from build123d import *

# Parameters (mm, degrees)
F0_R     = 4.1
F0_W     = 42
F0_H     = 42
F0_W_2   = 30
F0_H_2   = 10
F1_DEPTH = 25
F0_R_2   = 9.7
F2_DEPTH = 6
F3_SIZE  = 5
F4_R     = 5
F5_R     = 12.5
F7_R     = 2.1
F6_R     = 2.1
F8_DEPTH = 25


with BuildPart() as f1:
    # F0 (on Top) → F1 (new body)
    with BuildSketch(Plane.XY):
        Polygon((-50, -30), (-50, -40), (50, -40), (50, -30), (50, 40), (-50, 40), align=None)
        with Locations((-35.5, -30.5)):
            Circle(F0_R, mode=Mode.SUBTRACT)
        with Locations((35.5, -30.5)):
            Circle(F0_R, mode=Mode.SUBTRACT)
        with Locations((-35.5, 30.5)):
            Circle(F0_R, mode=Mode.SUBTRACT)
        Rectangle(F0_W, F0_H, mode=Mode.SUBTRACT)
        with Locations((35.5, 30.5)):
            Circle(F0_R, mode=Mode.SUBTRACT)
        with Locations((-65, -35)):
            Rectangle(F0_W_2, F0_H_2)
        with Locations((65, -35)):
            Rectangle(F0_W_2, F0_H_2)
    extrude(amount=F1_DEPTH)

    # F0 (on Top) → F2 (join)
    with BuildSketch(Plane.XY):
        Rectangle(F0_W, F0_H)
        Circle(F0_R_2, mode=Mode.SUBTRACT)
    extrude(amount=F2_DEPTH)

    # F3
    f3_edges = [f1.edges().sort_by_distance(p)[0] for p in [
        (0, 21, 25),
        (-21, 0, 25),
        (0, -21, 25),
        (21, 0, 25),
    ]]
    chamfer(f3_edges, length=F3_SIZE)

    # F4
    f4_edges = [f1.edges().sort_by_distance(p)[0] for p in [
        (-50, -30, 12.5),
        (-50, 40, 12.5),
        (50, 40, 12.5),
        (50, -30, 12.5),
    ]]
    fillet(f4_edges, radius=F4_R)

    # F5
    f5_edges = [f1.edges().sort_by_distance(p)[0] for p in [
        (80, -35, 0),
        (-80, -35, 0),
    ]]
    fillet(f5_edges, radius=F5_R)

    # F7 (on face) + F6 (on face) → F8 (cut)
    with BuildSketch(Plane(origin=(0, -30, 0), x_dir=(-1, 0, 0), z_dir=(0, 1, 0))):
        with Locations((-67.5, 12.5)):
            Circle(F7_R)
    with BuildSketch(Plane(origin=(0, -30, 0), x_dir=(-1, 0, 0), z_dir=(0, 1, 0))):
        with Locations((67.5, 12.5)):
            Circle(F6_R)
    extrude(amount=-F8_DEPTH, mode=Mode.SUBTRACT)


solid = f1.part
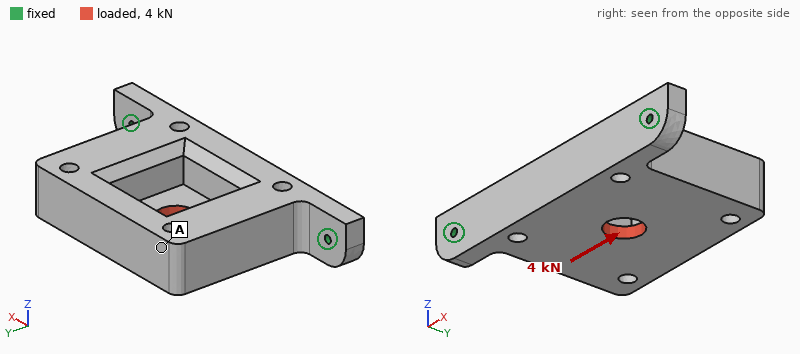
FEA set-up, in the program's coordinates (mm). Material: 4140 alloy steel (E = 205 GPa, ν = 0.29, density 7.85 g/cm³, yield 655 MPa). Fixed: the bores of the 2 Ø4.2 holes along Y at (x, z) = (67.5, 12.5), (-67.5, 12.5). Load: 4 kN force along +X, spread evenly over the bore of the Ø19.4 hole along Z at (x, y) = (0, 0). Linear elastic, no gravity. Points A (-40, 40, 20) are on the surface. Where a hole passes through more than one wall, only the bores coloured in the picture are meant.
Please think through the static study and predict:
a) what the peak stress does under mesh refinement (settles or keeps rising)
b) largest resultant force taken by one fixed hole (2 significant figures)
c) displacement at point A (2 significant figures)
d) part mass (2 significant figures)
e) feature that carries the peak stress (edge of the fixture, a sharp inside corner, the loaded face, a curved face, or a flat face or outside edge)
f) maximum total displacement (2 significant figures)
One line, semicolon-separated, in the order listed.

keeps rising; 2.3 kN; 8.0 µm; 1.3 kg; edge of the fixture; 8.9 µm
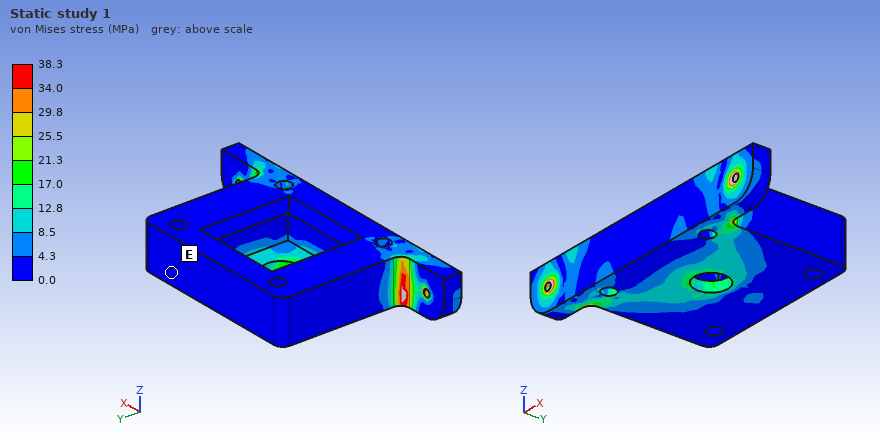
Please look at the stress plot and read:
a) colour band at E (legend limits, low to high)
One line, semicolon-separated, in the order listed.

0.0 to 4.3 MPa
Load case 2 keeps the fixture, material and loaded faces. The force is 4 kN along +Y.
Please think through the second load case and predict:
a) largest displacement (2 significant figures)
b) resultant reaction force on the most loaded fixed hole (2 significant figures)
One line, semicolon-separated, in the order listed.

64 µm; 2.3 kN
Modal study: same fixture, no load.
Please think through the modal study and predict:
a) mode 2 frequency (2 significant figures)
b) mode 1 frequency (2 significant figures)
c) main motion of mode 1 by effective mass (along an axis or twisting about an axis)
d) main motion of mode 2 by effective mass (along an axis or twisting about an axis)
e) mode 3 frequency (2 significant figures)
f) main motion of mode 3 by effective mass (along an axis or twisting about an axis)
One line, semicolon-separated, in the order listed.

3100 Hz; 700 Hz; along Z; along Y; 3200 Hz; along X
